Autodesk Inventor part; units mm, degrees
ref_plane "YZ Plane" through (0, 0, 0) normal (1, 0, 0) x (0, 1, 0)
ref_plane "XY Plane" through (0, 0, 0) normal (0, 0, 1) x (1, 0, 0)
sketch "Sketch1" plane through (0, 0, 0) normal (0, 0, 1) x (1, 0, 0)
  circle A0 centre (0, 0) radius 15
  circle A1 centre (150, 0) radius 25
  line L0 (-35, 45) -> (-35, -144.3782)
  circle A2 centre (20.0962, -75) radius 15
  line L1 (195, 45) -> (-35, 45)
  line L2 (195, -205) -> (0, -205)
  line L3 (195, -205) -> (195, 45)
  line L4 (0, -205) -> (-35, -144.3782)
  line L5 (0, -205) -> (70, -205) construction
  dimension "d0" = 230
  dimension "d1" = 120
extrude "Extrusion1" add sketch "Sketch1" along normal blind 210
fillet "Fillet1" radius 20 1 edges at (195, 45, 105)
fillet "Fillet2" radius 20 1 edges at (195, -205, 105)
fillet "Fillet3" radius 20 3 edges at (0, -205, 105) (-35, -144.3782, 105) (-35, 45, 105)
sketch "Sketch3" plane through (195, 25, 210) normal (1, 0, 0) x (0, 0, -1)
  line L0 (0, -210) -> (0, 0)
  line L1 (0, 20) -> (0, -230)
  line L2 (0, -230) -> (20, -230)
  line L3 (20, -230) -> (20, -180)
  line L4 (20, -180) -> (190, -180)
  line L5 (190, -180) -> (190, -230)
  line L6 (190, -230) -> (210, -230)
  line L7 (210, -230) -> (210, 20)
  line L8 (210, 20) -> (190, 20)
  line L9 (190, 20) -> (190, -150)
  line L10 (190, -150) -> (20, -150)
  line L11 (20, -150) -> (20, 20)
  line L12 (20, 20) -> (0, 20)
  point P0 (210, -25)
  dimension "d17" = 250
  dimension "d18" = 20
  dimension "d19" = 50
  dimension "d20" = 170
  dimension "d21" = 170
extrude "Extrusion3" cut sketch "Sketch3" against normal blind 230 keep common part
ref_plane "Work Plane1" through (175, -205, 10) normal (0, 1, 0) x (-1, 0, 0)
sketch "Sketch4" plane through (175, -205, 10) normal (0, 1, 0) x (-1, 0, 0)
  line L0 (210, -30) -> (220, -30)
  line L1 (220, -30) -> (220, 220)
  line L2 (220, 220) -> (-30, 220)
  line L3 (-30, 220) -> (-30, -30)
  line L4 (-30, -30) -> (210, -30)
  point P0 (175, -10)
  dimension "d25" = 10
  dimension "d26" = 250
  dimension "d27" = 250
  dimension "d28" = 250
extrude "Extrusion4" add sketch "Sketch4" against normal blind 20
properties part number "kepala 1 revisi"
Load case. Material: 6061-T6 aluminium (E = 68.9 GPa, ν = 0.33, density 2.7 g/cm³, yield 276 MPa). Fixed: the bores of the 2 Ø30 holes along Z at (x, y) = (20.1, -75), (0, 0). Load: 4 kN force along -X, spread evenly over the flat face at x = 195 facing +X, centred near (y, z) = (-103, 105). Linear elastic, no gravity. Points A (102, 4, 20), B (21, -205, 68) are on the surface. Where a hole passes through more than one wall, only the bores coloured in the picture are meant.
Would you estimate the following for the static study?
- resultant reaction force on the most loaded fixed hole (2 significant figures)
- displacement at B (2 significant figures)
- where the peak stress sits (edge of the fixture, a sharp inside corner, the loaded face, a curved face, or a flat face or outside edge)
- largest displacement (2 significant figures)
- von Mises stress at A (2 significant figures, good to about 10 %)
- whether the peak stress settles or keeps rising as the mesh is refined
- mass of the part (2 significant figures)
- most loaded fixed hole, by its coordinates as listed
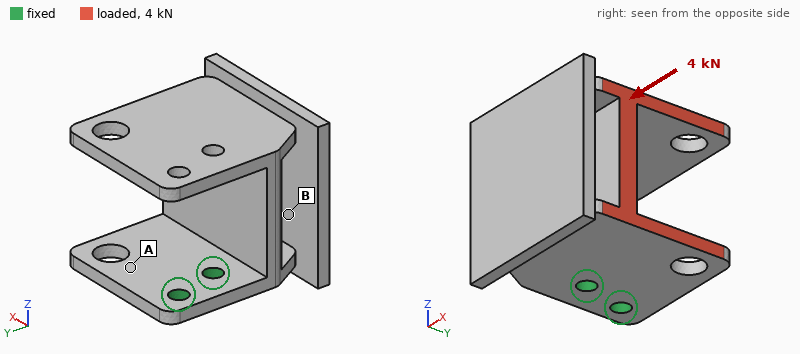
4.5 kN
0.083 mm
edge of the fixture
0.40 mm
5.3 MPa
keeps rising
12 kg
(20.1, -75)
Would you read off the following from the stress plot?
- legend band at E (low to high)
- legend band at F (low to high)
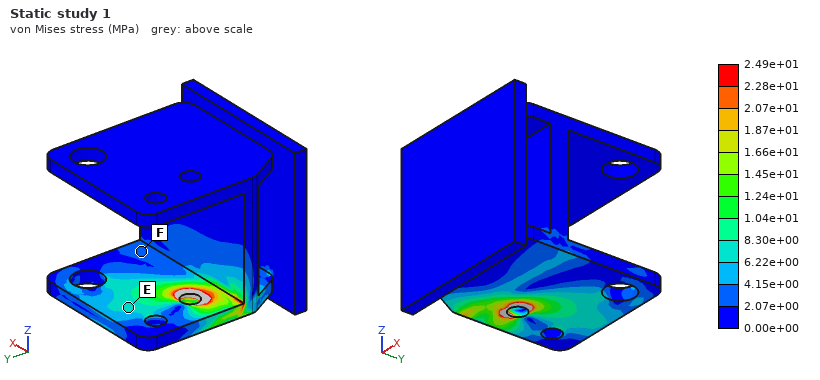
6.22e+00 to 8.30e+00 MPa
2.07e+00 to 4.15e+00 MPa
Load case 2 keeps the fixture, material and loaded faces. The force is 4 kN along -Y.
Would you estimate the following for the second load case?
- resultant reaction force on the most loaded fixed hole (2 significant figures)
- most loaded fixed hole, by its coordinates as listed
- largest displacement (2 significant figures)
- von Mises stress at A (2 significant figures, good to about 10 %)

7.6 kN
(20.1, -75)
0.77 mm
7.8 MPa
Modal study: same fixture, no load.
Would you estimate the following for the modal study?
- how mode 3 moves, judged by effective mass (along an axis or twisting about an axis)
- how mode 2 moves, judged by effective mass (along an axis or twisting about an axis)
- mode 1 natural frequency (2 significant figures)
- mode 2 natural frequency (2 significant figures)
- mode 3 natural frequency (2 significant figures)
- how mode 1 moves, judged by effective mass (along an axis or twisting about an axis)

along Z
along X
110 Hz
170 Hz
480 Hz
along Y
